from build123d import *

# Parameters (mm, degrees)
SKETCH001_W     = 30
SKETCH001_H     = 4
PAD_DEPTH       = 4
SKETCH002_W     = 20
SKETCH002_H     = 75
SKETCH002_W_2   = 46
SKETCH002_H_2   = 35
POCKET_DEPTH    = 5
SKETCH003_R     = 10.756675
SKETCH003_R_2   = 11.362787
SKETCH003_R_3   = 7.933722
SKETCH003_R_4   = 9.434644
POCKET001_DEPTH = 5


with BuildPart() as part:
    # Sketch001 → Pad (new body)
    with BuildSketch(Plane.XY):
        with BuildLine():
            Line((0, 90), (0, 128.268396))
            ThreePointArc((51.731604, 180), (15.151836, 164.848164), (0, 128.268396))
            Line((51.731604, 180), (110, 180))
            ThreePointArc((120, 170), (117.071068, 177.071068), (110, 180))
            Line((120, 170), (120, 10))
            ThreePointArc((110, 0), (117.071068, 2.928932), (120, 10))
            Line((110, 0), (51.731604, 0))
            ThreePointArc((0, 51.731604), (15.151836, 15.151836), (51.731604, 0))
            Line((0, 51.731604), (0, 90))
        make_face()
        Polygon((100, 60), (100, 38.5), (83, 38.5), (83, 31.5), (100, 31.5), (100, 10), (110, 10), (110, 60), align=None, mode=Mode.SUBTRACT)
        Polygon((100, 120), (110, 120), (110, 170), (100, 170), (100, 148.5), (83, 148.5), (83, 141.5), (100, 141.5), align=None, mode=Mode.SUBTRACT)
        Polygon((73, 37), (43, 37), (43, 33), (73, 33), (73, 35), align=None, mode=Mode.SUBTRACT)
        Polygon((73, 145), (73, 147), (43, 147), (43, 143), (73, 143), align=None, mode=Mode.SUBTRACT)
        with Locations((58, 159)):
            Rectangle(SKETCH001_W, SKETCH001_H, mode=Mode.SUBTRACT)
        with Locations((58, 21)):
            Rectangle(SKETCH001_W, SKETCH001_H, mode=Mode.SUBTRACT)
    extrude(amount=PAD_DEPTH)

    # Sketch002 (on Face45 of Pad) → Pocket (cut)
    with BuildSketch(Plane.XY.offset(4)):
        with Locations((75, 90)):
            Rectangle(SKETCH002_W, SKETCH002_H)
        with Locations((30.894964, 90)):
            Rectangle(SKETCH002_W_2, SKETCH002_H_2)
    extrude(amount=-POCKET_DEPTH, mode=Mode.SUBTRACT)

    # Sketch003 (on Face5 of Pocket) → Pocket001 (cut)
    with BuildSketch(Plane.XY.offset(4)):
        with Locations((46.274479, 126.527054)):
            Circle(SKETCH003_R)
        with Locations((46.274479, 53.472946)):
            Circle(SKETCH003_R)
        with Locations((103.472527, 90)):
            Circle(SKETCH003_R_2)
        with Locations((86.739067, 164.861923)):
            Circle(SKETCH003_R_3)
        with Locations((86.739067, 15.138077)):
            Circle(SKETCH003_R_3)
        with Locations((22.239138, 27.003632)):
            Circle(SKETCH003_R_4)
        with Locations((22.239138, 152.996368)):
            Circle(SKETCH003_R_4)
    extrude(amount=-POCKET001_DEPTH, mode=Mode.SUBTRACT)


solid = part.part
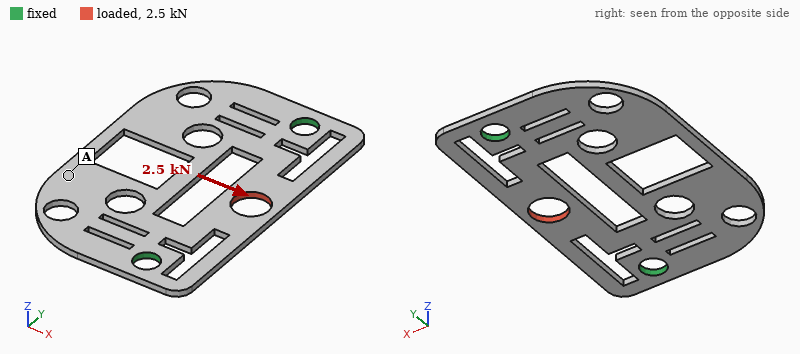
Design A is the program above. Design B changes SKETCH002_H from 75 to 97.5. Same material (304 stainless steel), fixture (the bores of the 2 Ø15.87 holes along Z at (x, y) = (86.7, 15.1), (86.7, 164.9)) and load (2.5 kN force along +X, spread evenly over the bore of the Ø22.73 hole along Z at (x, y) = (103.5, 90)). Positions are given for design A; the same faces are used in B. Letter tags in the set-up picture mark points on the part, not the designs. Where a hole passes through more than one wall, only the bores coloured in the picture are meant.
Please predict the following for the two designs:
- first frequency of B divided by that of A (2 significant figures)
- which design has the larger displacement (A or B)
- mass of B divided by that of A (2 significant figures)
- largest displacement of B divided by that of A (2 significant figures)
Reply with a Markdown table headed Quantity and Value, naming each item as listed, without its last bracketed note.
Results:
| Quantity | Value |
|---|---|
| first frequency of B divided by that of A | 0.95 |
| which design has the larger displacement | B |
| mass of B divided by that of A | 0.97 |
| largest displacement of B divided by that of A | 1.8 |
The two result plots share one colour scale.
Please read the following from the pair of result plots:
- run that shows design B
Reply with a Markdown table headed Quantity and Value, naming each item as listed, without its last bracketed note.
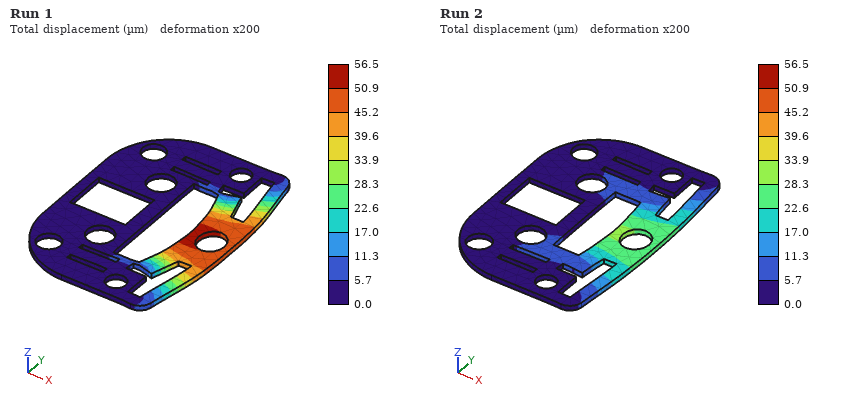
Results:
| Quantity | Value |
|---|---|
| run that shows design B | Run 1 |
